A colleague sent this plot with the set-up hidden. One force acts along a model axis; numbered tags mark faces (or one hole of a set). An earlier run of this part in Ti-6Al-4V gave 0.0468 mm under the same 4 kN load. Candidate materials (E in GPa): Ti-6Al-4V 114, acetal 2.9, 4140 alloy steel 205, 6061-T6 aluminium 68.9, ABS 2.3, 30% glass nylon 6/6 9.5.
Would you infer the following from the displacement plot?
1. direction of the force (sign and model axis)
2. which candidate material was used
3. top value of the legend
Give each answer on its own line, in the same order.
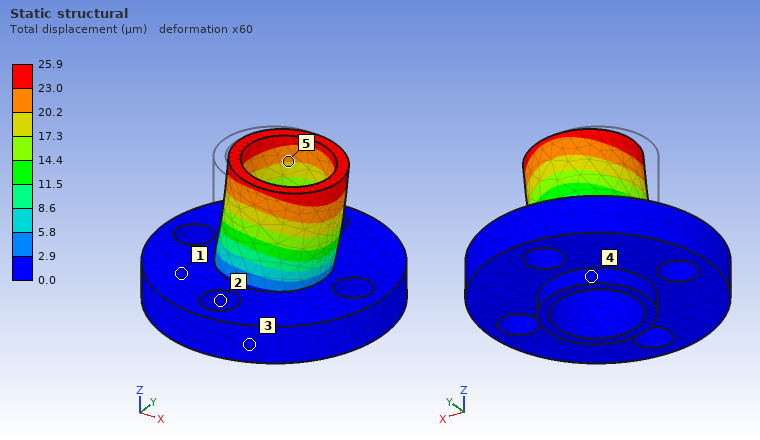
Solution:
+X
4140 alloy steel
25.9 µm
